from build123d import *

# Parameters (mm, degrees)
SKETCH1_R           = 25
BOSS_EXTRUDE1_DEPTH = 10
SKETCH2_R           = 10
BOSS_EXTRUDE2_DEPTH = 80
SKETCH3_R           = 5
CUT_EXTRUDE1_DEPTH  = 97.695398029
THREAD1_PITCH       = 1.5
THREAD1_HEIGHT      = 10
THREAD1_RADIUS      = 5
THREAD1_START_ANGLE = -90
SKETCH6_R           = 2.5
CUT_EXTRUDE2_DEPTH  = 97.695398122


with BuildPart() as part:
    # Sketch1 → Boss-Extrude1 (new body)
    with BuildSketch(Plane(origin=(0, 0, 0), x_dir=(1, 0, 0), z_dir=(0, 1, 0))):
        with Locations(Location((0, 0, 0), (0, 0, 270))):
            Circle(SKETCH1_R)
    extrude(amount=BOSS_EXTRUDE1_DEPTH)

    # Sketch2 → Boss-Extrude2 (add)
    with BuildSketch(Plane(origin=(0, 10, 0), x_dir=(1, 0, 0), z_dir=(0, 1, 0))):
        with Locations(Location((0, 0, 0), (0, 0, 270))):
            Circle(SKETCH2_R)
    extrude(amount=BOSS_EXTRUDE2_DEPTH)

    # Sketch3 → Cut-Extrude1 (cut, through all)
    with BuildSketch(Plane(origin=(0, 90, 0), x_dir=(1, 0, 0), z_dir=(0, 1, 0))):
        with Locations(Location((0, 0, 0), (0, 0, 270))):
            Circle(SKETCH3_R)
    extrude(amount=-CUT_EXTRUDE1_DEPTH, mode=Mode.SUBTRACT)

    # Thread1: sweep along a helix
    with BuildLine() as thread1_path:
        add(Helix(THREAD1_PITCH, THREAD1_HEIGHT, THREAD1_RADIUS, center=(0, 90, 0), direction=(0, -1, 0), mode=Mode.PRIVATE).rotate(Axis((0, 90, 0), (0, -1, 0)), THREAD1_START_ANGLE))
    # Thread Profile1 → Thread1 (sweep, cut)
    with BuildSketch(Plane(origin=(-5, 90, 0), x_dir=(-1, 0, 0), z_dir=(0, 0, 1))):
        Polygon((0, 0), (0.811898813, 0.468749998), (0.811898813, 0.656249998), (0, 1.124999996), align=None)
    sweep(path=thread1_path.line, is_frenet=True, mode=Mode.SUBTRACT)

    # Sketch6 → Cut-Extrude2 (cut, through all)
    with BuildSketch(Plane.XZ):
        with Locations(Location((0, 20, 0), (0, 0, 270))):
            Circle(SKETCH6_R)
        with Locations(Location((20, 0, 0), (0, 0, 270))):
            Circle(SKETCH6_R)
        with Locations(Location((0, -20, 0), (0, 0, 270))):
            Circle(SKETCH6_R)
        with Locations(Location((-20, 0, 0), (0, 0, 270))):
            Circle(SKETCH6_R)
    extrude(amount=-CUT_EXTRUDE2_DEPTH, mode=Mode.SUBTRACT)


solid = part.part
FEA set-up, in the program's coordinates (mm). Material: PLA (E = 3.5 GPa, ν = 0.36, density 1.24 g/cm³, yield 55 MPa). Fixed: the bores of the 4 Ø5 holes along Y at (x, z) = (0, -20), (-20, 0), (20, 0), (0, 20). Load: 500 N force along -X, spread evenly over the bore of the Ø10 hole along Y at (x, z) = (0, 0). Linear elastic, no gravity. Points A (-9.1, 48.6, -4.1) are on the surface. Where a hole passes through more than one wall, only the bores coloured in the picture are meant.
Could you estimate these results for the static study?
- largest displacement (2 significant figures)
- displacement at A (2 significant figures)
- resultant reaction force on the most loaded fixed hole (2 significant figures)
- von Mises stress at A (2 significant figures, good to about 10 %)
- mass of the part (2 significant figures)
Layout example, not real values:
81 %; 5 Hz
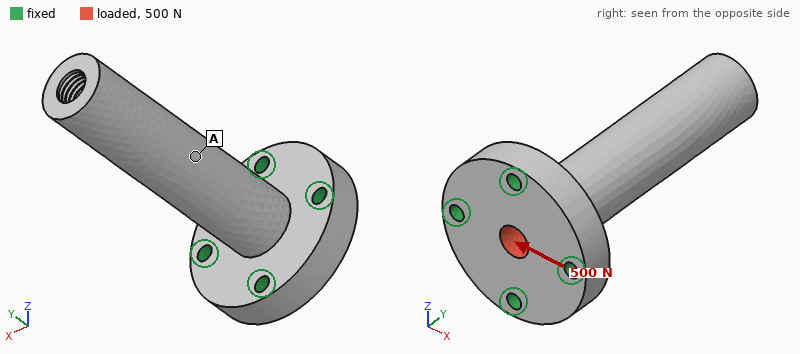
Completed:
1.3 mm; 0.57 mm; 510 N; 3.9 MPa; 46 g
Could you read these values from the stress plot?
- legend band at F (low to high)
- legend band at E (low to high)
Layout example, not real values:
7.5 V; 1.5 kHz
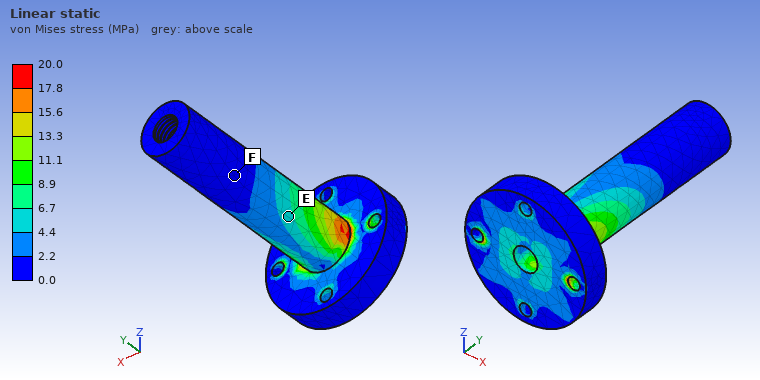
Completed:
0.0 to 2.2 MPa; 4.4 to 6.7 MPa
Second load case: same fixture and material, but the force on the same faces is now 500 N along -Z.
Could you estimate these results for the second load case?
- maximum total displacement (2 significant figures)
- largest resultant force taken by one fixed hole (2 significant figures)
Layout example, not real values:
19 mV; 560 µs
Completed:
1.3 mm; 510 N
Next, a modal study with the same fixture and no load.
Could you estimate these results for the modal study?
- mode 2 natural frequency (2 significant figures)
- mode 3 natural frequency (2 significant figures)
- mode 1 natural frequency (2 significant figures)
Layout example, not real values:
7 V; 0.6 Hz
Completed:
670 Hz; 3100 Hz; 670 Hz
